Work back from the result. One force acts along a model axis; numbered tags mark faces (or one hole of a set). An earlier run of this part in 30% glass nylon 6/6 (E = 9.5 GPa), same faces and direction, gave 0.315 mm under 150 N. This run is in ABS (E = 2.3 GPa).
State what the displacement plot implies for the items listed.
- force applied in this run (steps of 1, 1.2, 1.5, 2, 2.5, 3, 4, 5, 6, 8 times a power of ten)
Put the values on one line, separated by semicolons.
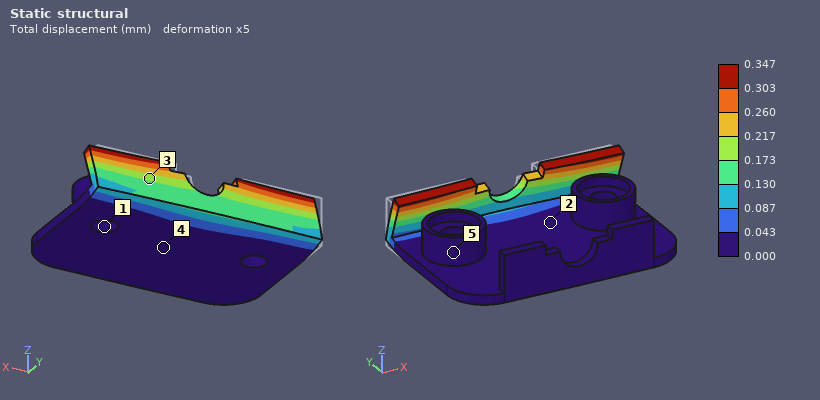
40 N
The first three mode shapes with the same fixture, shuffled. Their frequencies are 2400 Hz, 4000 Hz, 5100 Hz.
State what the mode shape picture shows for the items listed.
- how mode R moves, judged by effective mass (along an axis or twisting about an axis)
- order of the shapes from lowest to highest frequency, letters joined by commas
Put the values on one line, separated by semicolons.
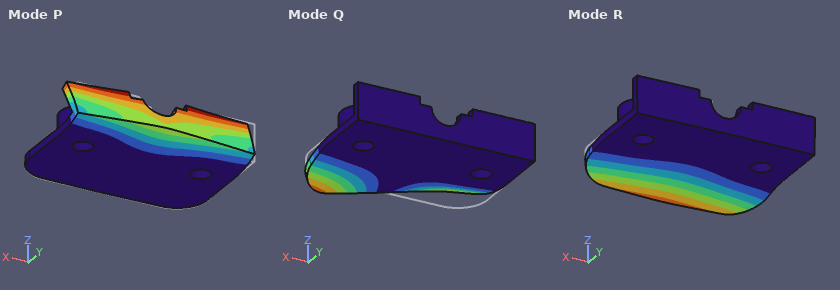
along Z; R, Q, P
